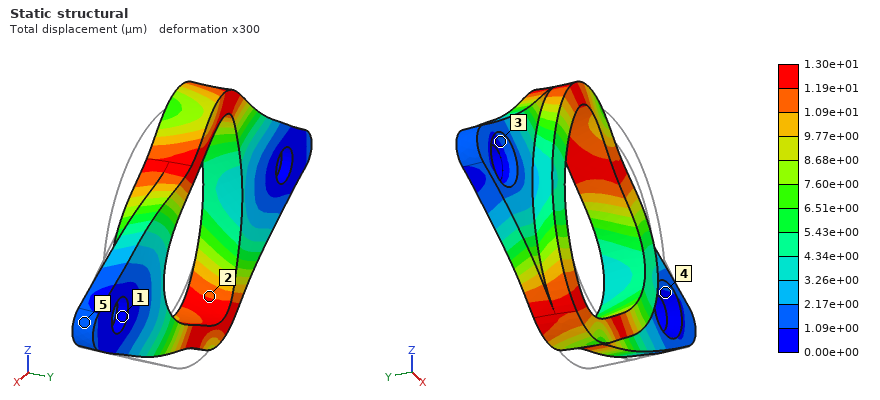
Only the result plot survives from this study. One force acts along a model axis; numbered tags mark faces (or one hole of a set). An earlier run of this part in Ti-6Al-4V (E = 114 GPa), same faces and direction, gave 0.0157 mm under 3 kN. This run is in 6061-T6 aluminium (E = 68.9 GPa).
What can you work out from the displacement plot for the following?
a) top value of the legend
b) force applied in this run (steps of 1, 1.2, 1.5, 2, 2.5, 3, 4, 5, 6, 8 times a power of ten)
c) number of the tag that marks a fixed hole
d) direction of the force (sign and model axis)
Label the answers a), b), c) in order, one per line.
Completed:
a) 1.30e+01 µm
b) 1.5 kN
c) 1
d) -X
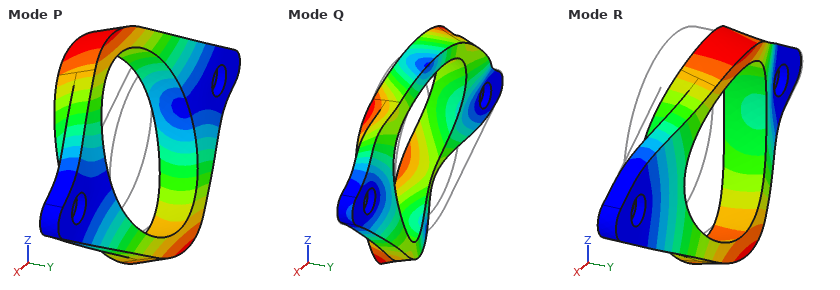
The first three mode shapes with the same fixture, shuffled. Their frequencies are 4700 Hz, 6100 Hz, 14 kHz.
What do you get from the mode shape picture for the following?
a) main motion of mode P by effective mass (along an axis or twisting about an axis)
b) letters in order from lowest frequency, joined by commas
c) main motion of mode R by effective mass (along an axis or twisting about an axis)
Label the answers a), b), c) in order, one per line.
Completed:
a) twisting about X
b) P, R, Q
c) along Y
